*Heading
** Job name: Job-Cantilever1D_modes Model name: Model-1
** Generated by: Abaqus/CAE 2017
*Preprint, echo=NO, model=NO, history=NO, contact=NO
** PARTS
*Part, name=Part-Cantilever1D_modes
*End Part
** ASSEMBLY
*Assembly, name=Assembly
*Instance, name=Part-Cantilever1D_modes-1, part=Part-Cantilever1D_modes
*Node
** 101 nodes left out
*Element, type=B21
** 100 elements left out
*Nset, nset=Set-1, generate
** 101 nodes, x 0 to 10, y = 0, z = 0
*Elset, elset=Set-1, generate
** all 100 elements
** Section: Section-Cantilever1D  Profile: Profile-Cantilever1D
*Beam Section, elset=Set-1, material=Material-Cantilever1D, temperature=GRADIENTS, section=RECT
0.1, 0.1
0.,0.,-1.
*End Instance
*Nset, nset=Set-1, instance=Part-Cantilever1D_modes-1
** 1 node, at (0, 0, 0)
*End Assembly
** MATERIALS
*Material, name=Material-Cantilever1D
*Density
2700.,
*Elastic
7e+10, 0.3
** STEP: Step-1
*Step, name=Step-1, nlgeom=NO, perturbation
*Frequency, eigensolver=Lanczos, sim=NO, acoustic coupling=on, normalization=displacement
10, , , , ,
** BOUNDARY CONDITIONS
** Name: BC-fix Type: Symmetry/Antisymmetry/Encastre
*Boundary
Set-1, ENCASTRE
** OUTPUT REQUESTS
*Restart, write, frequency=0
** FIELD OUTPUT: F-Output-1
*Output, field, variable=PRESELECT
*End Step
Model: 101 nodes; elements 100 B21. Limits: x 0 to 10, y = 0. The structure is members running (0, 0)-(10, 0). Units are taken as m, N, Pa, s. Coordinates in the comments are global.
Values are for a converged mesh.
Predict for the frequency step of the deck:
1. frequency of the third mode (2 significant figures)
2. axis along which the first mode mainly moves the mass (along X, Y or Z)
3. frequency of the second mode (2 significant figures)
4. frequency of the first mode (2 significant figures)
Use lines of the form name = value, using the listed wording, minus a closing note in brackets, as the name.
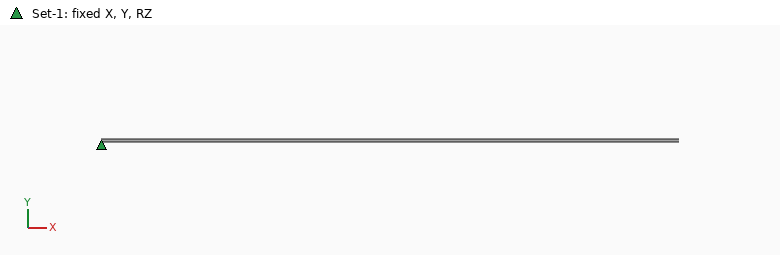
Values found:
frequency of the third mode = 14 Hz
axis along which the first mode mainly moves the mass = along Y
frequency of the second mode = 5.2 Hz
frequency of the first mode = 0.82 Hz
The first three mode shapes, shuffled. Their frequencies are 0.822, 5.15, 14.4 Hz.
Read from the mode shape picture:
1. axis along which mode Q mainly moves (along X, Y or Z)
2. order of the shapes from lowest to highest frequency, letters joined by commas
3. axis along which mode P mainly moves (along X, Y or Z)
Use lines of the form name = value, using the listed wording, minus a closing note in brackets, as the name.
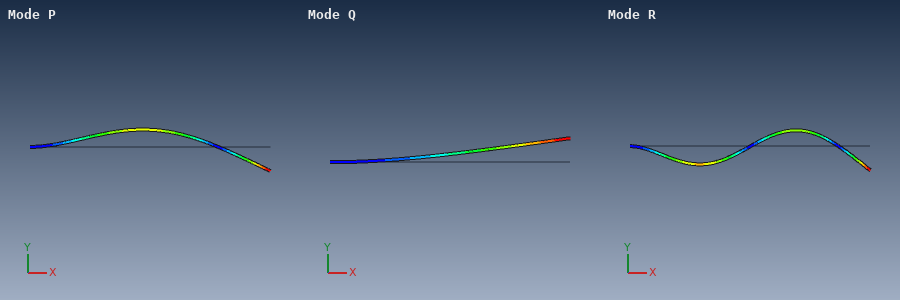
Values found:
axis along which mode Q mainly moves = along Y
order of the shapes from lowest to highest frequency, letters joined by commas = Q, P, R
axis along which mode P mainly moves = along Y
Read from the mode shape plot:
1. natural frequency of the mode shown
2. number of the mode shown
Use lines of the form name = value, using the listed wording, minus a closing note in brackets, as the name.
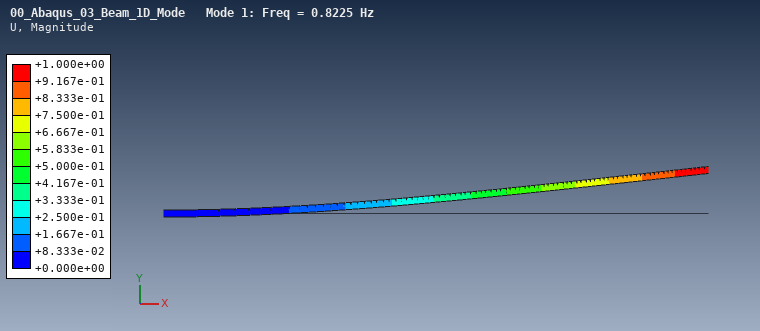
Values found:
natural frequency of the mode shown = 0.8225 Hz
number of the mode shown = 1
